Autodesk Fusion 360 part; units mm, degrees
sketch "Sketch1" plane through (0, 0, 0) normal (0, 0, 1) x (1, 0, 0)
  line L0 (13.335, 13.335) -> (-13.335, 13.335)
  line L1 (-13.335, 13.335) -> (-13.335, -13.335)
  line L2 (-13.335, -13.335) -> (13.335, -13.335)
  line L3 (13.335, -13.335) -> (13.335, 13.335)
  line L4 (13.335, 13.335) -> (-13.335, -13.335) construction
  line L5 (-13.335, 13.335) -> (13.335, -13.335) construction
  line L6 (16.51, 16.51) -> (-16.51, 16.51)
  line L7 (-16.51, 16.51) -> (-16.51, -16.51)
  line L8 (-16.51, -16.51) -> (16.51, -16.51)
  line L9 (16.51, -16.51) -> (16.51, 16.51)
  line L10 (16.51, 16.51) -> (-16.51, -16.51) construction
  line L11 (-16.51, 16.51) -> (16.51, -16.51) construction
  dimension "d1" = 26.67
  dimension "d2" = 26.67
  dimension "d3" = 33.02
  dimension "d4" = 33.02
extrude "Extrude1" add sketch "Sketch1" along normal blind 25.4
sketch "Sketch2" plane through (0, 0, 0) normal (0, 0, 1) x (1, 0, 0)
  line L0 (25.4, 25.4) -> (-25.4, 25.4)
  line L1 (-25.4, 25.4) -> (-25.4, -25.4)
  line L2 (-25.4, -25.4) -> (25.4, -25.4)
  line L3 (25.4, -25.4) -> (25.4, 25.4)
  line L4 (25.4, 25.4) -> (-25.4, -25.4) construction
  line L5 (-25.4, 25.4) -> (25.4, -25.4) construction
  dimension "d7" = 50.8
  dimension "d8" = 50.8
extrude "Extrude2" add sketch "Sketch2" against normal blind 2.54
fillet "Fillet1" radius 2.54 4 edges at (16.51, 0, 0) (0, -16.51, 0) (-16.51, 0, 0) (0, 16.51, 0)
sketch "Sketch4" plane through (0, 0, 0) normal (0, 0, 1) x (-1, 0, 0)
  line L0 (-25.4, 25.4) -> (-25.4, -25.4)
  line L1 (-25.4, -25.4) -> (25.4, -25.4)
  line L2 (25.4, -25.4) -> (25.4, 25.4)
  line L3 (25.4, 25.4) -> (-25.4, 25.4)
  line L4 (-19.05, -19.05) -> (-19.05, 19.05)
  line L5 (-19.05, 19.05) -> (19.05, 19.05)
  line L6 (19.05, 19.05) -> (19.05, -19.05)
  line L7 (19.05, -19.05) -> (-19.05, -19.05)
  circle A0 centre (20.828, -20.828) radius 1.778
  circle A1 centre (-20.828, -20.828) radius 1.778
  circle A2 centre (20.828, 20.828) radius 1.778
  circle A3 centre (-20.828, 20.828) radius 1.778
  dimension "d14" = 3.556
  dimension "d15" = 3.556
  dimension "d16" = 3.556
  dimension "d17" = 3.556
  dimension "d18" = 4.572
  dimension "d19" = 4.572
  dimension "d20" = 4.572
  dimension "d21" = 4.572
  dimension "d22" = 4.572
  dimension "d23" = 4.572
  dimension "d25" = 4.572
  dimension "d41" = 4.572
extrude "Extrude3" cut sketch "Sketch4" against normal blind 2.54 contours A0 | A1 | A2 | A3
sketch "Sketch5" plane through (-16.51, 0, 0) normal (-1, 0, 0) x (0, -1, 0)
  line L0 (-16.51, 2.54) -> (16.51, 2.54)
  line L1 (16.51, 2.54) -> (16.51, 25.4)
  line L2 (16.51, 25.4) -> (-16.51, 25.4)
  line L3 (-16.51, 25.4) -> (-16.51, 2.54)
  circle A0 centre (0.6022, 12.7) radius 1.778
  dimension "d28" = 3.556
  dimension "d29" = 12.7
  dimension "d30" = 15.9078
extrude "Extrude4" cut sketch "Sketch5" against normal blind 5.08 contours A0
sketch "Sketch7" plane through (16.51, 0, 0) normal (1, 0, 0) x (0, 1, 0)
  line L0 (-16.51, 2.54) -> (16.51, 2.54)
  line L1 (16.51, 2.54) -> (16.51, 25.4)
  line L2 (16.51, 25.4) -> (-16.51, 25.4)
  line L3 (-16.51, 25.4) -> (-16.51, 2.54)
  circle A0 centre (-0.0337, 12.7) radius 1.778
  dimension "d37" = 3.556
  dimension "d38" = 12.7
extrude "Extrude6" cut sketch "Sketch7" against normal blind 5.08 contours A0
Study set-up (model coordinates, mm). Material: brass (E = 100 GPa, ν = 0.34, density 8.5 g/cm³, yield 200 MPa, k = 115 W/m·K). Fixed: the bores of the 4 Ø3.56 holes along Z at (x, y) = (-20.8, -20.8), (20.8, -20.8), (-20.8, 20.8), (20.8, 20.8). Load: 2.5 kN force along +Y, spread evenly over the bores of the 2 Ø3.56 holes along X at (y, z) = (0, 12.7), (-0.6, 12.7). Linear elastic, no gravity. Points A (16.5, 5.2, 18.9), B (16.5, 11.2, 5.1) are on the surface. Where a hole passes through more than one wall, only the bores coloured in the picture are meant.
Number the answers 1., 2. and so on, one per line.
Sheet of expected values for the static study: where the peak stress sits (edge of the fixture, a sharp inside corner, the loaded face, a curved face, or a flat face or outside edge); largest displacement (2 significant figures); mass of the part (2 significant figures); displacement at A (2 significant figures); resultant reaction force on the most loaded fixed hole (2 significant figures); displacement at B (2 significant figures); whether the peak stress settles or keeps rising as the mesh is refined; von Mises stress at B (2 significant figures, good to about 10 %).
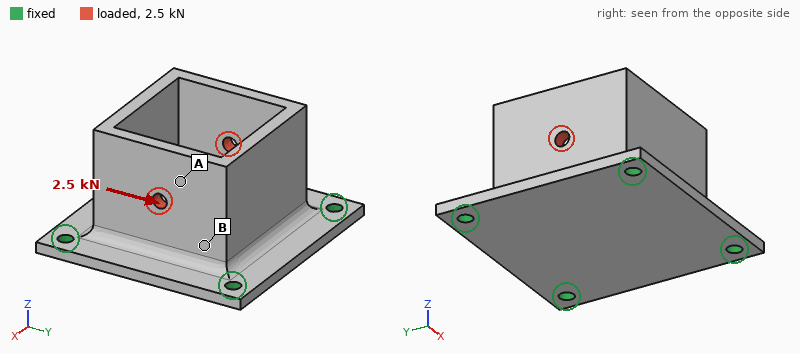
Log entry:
1. edge of the fixture
2. 26 µm
3. 140 g
4. 19 µm
5. 830 N
6. 9.9 µm
7. keeps rising
8. 26 MPa
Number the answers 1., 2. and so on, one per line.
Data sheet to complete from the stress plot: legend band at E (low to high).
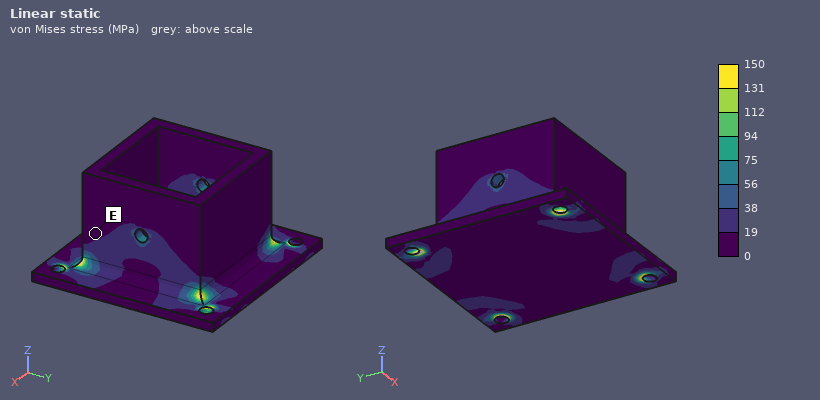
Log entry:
1. 0 to 19 MPa
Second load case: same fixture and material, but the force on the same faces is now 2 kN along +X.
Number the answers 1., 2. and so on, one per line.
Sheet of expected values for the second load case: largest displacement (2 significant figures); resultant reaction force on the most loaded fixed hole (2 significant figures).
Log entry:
1. 46 µm
2. 690 N
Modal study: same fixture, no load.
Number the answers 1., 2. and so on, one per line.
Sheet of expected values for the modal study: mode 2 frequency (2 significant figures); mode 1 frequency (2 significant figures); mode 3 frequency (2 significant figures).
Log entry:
1. 5200 Hz
2. 5200 Hz
3. 5200 Hz
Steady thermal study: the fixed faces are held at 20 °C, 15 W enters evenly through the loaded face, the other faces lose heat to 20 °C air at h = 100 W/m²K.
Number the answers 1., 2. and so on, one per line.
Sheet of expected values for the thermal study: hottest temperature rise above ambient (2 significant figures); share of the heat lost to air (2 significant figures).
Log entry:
1. 14 K
2. 42 %
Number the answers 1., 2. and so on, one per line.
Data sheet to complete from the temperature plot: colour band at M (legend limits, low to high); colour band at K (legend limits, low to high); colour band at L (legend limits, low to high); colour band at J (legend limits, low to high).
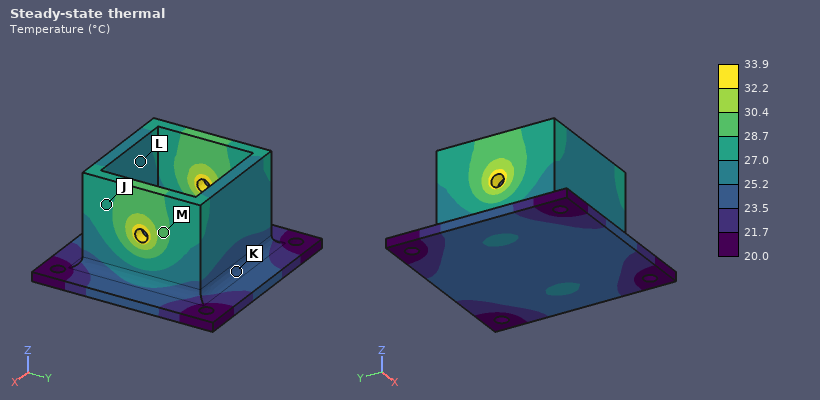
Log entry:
1. 28.7 to 30.4 °C
2. 23.5 to 25.2 °C
3. 25.2 to 27.0 °C
4. 27.0 to 28.7 °C
